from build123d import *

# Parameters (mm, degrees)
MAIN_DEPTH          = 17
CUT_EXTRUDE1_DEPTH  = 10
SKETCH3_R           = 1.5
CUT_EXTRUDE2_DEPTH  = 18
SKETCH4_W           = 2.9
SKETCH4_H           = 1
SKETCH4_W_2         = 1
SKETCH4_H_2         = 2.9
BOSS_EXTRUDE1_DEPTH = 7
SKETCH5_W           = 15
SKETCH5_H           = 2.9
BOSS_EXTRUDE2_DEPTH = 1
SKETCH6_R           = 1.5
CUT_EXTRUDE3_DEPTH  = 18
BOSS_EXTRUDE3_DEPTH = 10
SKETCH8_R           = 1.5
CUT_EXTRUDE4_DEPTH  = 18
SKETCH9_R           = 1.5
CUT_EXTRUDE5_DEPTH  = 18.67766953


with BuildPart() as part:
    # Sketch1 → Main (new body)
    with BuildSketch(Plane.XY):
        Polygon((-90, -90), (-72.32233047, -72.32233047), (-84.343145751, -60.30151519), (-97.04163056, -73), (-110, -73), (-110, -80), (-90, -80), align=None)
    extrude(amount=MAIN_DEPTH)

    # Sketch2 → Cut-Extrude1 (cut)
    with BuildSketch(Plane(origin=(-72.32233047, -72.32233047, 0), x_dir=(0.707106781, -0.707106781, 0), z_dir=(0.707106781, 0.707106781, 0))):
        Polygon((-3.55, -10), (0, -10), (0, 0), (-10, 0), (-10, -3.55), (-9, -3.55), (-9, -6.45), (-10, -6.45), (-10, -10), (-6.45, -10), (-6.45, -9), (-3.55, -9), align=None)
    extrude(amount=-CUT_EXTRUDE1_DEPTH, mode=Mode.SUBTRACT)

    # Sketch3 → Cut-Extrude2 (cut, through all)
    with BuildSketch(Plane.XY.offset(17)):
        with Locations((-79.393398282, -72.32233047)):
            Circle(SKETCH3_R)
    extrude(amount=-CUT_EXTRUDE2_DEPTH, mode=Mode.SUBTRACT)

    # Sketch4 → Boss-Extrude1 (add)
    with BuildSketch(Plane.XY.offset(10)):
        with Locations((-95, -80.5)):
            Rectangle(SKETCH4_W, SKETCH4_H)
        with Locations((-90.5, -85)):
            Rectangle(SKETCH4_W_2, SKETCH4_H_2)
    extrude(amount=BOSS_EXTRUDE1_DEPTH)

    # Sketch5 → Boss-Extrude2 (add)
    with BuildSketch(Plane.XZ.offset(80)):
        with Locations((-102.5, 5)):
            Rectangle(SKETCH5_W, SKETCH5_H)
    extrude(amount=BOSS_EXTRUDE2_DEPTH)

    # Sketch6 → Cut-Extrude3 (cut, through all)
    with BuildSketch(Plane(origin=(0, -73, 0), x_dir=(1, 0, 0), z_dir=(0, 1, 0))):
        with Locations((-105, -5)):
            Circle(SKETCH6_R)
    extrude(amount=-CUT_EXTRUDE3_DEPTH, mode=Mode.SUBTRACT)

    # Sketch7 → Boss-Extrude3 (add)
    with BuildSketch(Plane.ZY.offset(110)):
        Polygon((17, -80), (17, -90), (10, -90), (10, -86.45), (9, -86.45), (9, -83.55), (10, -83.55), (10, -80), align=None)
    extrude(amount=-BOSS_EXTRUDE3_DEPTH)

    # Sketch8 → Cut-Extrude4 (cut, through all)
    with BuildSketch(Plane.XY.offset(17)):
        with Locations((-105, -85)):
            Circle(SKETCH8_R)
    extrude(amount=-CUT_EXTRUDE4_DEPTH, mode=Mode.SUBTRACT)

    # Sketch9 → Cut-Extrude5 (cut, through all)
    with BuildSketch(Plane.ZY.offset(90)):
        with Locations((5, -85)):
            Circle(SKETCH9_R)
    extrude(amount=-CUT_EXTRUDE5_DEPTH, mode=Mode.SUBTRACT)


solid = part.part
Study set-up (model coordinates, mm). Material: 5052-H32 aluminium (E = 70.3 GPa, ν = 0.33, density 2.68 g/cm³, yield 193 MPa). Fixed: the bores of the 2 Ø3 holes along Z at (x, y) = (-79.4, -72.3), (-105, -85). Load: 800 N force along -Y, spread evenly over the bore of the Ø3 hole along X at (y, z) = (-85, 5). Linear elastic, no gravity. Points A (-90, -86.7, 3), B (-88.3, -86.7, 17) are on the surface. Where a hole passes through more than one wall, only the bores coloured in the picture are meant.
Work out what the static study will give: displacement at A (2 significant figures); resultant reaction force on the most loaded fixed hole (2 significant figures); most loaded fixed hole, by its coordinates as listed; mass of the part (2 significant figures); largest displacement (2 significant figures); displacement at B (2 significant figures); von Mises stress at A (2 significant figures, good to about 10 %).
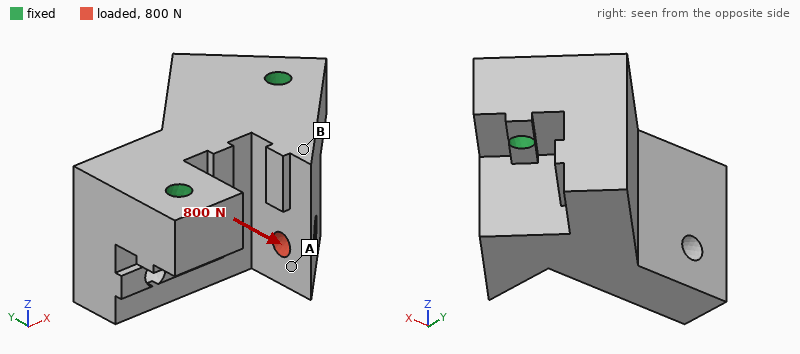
18 µm
540 N
(-79.4, -72.3)
19 g
21 µm
11 µm
13 MPa
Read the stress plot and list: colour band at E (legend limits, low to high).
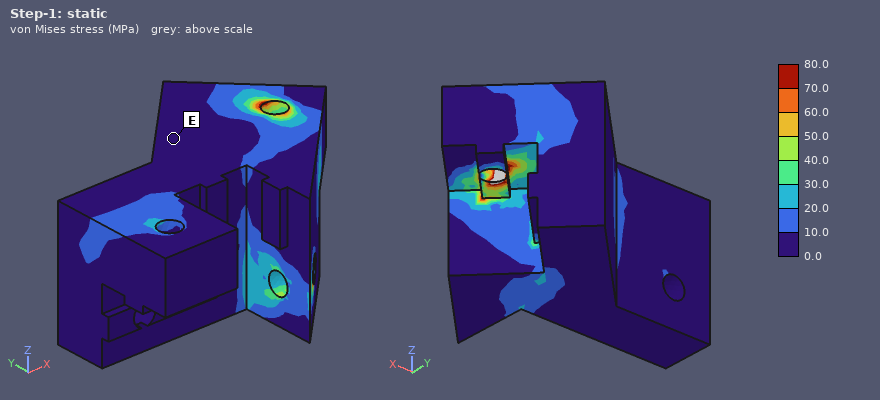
0.0 to 10.0 MPa
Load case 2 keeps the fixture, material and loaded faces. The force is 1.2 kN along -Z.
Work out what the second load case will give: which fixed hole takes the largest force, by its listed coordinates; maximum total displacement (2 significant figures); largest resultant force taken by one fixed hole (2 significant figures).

(-79.4, -72.3)
43 µm
830 N
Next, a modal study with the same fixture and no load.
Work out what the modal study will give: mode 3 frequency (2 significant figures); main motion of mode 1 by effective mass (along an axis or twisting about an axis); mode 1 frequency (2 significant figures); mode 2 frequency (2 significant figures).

25 kHz
along Y
12 kHz
20 kHz
